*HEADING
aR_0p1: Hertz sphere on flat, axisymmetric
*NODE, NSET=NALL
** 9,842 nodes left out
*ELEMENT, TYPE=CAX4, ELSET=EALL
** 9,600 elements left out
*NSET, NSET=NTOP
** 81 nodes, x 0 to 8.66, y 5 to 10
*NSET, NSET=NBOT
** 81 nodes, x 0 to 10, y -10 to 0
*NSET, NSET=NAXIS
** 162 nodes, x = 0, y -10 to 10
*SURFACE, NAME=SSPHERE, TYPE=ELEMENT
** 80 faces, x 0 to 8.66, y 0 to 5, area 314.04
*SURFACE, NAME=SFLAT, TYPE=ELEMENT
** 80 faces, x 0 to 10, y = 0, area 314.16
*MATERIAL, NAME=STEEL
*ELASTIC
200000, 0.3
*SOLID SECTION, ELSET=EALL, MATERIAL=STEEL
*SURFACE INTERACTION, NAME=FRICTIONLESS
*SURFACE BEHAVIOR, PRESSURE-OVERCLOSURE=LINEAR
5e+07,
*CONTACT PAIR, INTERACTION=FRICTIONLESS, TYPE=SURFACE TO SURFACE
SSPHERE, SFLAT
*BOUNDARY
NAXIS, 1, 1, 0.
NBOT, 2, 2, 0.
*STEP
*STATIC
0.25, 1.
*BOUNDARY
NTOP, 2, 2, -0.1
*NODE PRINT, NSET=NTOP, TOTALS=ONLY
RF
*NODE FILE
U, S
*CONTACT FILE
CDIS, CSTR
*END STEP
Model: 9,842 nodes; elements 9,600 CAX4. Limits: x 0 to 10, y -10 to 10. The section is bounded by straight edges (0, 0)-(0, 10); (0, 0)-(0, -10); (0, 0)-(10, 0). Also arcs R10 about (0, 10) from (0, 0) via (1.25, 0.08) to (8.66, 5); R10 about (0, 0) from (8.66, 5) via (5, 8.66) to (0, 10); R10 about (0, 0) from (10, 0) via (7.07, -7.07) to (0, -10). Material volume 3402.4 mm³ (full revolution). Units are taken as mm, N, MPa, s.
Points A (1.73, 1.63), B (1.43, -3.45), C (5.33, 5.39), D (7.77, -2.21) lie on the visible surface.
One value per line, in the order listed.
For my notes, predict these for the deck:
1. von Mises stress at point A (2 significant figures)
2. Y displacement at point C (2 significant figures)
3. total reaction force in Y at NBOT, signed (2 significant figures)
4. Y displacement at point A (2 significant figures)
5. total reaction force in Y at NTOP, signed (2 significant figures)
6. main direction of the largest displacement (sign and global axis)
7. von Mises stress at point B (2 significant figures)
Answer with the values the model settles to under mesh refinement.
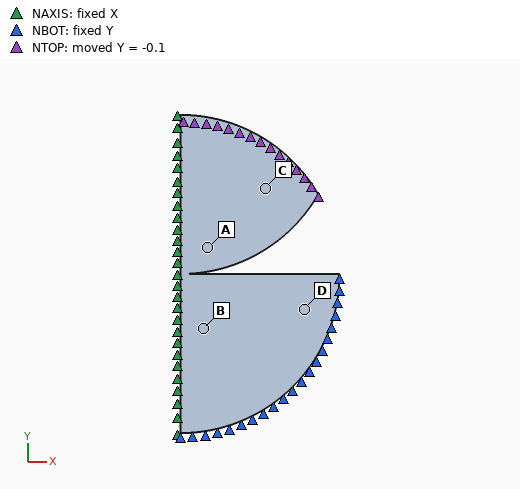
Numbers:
870 MPa
-0.099 mm
16000 N
-0.090 mm
-16000 N
-Y
510 MPa
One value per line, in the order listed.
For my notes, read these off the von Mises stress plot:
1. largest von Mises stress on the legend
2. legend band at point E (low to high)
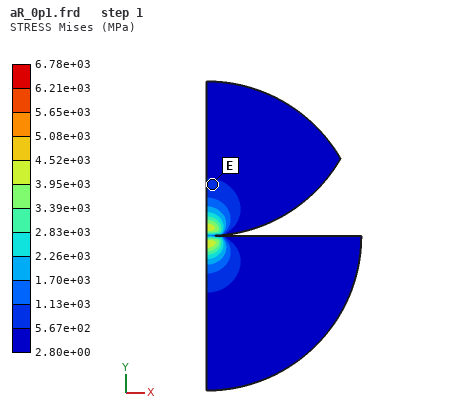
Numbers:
6.78e+03 MPa
5.67e+02 to 1.13e+03 MPa
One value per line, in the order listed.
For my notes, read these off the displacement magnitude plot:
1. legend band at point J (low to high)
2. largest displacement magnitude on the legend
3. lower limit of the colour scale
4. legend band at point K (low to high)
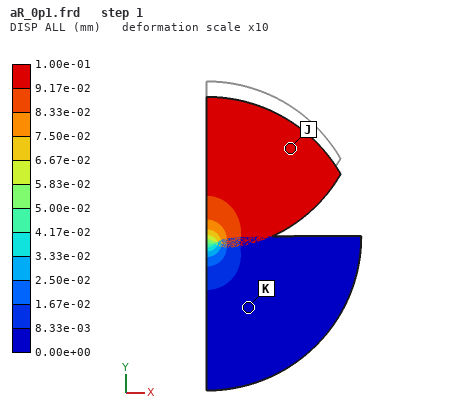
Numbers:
9.17e-02 to 1.00e-01 mm
1.00e-01 mm
0.00e+00 mm
0.00e+00 to 8.33e-03 mm
